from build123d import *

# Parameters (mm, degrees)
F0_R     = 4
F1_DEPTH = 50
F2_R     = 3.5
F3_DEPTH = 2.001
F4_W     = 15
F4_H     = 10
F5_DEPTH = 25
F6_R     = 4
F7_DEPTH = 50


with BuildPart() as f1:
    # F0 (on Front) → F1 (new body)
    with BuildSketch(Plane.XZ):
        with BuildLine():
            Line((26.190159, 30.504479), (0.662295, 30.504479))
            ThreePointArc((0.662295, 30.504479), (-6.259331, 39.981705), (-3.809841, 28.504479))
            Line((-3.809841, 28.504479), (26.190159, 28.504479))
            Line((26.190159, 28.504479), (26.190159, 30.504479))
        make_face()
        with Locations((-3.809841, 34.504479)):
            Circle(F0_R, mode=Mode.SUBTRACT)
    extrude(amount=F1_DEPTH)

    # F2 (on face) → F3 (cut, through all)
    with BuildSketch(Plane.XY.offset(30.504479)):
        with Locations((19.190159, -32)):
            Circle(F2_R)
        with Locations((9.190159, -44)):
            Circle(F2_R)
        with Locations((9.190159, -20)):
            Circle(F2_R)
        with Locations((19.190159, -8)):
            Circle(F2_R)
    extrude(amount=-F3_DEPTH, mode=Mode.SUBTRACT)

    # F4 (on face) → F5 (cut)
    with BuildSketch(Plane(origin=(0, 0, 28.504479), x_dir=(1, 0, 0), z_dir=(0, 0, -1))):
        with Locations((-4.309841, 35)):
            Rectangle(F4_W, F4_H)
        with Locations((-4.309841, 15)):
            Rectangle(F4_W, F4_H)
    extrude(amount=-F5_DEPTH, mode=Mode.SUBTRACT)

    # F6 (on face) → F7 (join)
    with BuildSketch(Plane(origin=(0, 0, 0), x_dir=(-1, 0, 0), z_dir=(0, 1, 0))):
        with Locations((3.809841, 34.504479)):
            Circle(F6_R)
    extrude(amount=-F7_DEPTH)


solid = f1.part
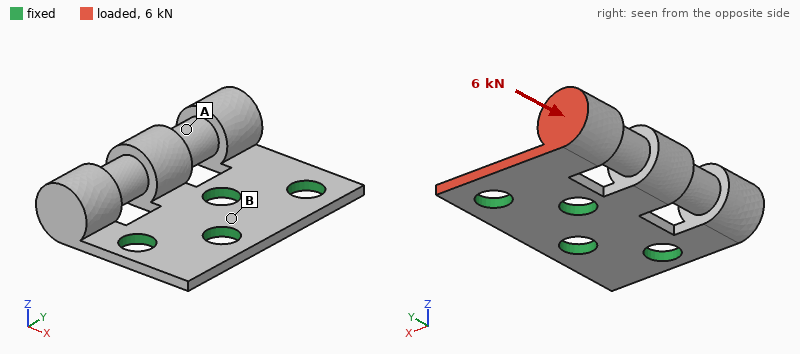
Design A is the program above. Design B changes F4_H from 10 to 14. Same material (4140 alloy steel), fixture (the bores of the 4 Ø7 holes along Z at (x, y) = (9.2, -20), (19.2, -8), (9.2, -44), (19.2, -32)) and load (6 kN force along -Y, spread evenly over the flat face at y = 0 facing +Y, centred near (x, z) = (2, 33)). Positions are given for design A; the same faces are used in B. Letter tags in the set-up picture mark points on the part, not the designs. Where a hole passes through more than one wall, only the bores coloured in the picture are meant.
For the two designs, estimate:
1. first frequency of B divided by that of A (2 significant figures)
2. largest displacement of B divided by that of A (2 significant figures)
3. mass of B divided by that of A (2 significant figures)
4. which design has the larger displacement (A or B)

0.91
1.4
0.91
B
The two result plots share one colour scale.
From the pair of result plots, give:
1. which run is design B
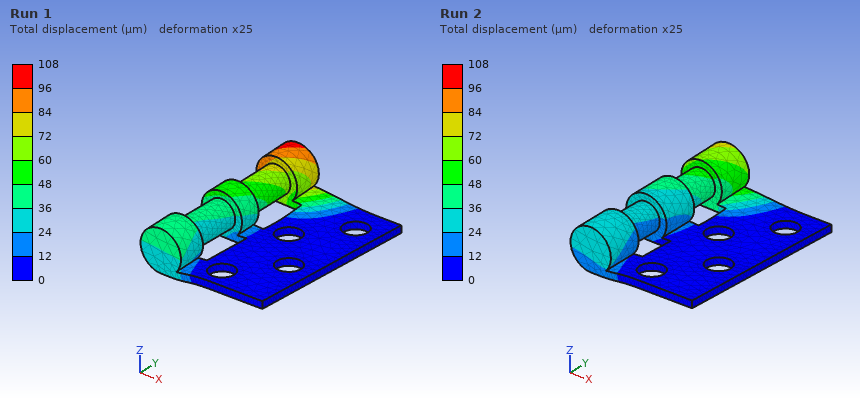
Run 1
